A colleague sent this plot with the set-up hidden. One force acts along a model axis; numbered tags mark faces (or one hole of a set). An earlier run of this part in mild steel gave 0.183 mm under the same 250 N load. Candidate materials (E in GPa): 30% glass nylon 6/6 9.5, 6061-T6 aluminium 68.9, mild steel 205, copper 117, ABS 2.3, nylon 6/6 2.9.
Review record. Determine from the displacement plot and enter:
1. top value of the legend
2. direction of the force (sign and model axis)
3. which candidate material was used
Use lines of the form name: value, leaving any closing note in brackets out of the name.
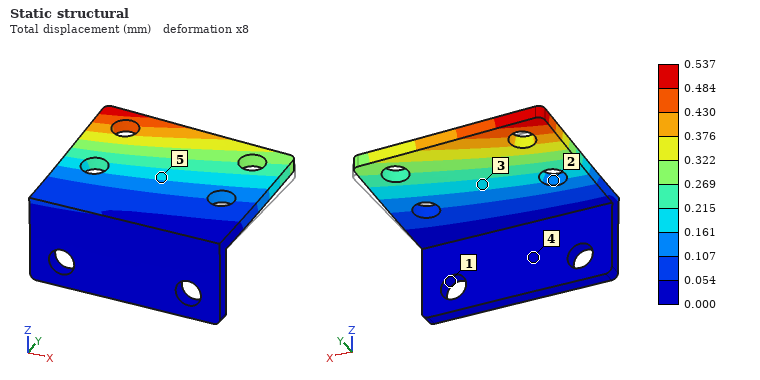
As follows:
top value of the legend: 0.537 mm
direction of the force: +Z
which candidate material was used: 6061-T6 aluminium
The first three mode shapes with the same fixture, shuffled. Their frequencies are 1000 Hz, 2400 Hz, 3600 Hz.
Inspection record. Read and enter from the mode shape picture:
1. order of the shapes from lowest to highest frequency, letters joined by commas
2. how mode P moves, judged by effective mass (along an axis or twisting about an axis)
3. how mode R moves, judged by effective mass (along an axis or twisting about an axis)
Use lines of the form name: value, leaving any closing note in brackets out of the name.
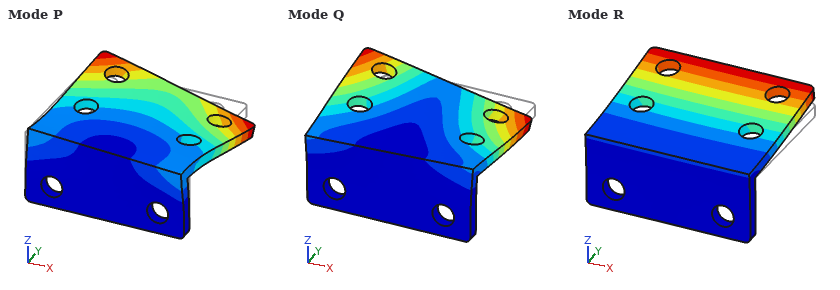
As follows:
order of the shapes from lowest to highest frequency, letters joined by commas: R, Q, P
how mode P moves, judged by effective mass: along X
how mode R moves, judged by effective mass: along Z
